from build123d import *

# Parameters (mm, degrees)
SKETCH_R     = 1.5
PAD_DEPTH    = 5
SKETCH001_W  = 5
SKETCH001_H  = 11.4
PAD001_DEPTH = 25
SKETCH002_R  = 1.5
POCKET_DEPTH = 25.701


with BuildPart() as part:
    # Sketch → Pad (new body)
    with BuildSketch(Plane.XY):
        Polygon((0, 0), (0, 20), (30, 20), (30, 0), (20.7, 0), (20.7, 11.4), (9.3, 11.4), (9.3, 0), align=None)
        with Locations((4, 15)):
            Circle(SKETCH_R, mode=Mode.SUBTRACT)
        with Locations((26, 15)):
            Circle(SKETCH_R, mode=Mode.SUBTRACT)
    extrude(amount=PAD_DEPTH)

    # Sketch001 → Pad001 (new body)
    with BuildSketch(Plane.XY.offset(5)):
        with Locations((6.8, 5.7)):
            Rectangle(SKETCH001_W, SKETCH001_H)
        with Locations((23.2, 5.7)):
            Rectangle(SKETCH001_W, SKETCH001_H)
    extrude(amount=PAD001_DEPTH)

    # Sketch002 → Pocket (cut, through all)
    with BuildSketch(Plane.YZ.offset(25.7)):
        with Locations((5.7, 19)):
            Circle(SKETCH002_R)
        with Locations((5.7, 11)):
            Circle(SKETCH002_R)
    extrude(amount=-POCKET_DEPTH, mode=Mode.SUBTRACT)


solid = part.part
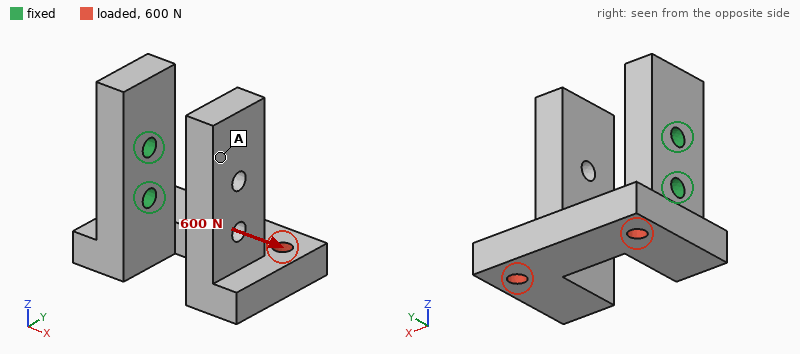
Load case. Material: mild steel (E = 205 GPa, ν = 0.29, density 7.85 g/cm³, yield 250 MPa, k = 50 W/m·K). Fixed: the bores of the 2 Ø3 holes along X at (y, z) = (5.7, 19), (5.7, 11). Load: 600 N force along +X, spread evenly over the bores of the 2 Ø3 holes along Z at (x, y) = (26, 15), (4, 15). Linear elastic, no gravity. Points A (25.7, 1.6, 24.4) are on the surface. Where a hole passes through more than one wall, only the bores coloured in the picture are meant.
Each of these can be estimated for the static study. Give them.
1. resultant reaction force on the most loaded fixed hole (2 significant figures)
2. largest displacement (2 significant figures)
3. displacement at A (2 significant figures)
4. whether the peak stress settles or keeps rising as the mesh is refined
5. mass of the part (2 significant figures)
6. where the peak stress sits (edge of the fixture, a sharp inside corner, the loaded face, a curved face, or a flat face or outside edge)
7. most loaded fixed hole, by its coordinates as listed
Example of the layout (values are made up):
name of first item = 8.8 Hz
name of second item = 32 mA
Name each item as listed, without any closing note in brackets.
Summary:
resultant reaction force on the most loaded fixed hole = 720 N
largest displacement = 56 µm
displacement at A = 44 µm
whether the peak stress settles or keeps rising as the mesh is refined = keeps rising
mass of the part = 39 g
where the peak stress sits = edge of the fixture
most loaded fixed hole, by its coordinates as listed = (5.7, 11)
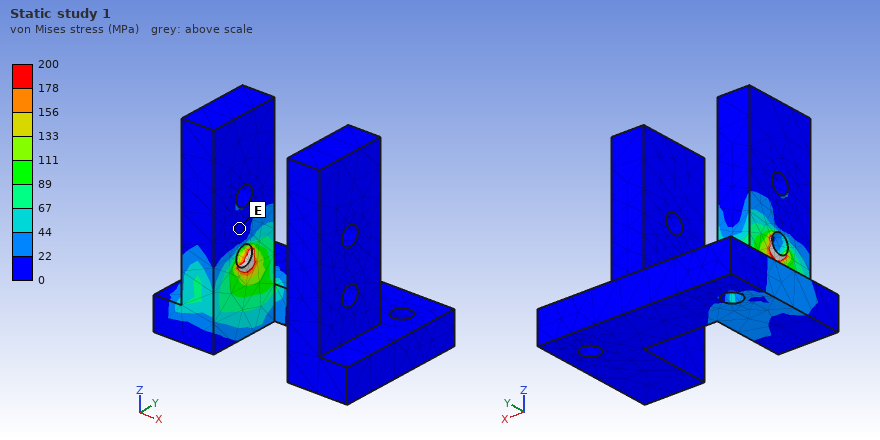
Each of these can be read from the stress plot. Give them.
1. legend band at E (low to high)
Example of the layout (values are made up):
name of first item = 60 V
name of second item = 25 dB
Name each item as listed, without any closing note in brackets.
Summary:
legend band at E = 0 to 22 MPa
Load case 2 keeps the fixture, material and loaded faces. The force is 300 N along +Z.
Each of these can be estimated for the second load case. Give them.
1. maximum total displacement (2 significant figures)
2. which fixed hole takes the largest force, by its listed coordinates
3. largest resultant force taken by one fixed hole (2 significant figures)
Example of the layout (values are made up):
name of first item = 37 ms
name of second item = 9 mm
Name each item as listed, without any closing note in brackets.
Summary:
maximum total displacement = 89 µm
which fixed hole takes the largest force, by its listed coordinates = (5.7, 11)
largest resultant force taken by one fixed hole = 320 N
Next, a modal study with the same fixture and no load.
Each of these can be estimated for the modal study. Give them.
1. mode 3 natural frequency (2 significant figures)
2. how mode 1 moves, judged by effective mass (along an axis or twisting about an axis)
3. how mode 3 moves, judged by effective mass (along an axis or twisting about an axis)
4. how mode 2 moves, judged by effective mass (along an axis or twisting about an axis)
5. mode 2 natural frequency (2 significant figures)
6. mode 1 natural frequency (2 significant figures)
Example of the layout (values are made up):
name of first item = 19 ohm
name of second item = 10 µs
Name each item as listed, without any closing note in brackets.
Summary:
mode 3 natural frequency = 3500 Hz
how mode 1 moves, judged by effective mass = along Z
how mode 3 moves, judged by effective mass = along Y
how mode 2 moves, judged by effective mass = along Y
mode 2 natural frequency = 1900 Hz
mode 1 natural frequency = 1600 Hz
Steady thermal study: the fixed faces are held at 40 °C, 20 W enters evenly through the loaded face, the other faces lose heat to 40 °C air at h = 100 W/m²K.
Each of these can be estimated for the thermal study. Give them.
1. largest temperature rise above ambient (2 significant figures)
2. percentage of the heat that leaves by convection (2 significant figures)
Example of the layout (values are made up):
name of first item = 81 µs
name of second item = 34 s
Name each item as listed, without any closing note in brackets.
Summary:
largest temperature rise above ambient = 76 K
percentage of the heat that leaves by convection = 54 %
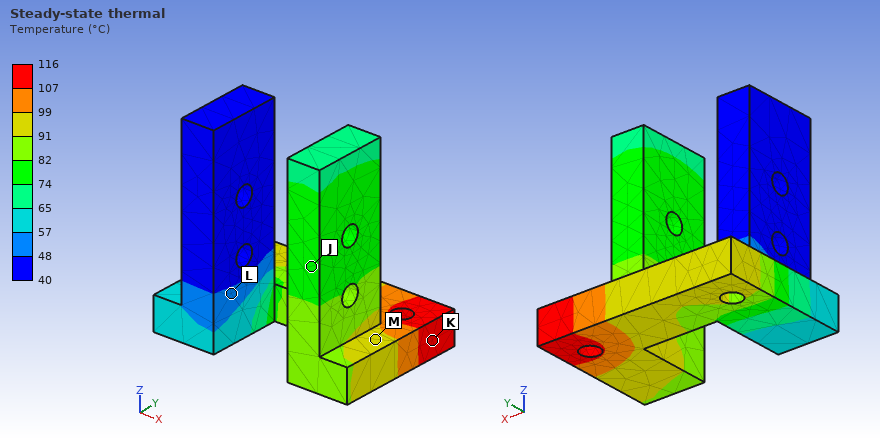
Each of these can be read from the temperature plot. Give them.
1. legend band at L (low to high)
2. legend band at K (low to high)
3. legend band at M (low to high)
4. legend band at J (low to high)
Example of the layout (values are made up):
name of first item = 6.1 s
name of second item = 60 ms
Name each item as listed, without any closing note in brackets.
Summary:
legend band at L = 48 to 57 °C
legend band at K = 107 to 116 °C
legend band at M = 91 to 99 °C
legend band at J = 74 to 82 °C
